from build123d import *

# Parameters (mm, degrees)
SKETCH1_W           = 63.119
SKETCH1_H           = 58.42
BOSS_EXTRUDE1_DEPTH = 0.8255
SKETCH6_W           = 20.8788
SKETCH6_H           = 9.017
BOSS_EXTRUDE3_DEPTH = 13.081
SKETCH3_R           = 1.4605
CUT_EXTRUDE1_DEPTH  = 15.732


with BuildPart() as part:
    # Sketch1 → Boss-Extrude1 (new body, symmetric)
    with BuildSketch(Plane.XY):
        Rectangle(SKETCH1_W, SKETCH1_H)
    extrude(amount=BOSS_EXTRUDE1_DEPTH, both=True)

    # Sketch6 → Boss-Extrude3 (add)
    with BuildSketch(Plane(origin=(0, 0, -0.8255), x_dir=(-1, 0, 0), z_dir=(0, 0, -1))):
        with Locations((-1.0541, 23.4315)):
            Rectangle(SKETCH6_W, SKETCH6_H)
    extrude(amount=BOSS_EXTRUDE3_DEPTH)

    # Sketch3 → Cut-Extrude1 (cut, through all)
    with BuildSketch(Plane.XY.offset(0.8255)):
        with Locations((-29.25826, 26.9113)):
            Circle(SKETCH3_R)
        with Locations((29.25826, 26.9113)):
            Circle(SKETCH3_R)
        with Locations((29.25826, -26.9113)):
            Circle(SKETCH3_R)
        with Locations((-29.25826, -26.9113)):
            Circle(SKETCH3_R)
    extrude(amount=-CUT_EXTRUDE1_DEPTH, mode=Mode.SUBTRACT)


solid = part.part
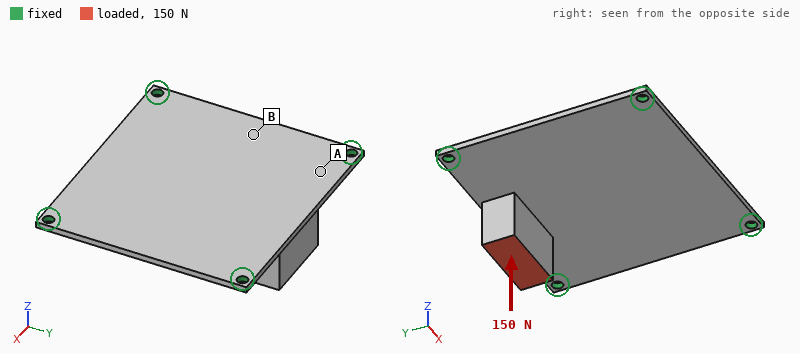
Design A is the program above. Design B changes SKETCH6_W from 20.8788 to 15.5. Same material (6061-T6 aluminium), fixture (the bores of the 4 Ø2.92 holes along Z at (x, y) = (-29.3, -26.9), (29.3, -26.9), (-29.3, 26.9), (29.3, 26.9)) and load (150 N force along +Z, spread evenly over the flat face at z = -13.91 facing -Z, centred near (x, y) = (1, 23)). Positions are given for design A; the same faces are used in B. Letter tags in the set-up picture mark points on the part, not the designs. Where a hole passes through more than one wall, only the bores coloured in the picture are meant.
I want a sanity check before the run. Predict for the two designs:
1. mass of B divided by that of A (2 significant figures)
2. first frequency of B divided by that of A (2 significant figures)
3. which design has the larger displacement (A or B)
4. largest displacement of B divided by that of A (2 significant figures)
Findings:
0.93
0.98
B
1.4
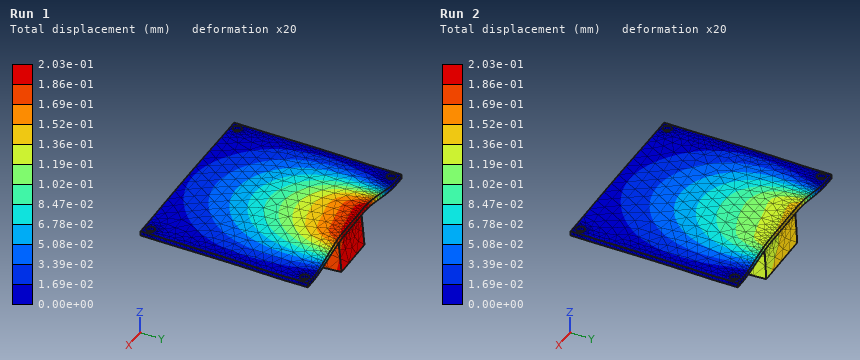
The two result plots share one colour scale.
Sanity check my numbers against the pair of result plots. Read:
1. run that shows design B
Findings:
Run 1
